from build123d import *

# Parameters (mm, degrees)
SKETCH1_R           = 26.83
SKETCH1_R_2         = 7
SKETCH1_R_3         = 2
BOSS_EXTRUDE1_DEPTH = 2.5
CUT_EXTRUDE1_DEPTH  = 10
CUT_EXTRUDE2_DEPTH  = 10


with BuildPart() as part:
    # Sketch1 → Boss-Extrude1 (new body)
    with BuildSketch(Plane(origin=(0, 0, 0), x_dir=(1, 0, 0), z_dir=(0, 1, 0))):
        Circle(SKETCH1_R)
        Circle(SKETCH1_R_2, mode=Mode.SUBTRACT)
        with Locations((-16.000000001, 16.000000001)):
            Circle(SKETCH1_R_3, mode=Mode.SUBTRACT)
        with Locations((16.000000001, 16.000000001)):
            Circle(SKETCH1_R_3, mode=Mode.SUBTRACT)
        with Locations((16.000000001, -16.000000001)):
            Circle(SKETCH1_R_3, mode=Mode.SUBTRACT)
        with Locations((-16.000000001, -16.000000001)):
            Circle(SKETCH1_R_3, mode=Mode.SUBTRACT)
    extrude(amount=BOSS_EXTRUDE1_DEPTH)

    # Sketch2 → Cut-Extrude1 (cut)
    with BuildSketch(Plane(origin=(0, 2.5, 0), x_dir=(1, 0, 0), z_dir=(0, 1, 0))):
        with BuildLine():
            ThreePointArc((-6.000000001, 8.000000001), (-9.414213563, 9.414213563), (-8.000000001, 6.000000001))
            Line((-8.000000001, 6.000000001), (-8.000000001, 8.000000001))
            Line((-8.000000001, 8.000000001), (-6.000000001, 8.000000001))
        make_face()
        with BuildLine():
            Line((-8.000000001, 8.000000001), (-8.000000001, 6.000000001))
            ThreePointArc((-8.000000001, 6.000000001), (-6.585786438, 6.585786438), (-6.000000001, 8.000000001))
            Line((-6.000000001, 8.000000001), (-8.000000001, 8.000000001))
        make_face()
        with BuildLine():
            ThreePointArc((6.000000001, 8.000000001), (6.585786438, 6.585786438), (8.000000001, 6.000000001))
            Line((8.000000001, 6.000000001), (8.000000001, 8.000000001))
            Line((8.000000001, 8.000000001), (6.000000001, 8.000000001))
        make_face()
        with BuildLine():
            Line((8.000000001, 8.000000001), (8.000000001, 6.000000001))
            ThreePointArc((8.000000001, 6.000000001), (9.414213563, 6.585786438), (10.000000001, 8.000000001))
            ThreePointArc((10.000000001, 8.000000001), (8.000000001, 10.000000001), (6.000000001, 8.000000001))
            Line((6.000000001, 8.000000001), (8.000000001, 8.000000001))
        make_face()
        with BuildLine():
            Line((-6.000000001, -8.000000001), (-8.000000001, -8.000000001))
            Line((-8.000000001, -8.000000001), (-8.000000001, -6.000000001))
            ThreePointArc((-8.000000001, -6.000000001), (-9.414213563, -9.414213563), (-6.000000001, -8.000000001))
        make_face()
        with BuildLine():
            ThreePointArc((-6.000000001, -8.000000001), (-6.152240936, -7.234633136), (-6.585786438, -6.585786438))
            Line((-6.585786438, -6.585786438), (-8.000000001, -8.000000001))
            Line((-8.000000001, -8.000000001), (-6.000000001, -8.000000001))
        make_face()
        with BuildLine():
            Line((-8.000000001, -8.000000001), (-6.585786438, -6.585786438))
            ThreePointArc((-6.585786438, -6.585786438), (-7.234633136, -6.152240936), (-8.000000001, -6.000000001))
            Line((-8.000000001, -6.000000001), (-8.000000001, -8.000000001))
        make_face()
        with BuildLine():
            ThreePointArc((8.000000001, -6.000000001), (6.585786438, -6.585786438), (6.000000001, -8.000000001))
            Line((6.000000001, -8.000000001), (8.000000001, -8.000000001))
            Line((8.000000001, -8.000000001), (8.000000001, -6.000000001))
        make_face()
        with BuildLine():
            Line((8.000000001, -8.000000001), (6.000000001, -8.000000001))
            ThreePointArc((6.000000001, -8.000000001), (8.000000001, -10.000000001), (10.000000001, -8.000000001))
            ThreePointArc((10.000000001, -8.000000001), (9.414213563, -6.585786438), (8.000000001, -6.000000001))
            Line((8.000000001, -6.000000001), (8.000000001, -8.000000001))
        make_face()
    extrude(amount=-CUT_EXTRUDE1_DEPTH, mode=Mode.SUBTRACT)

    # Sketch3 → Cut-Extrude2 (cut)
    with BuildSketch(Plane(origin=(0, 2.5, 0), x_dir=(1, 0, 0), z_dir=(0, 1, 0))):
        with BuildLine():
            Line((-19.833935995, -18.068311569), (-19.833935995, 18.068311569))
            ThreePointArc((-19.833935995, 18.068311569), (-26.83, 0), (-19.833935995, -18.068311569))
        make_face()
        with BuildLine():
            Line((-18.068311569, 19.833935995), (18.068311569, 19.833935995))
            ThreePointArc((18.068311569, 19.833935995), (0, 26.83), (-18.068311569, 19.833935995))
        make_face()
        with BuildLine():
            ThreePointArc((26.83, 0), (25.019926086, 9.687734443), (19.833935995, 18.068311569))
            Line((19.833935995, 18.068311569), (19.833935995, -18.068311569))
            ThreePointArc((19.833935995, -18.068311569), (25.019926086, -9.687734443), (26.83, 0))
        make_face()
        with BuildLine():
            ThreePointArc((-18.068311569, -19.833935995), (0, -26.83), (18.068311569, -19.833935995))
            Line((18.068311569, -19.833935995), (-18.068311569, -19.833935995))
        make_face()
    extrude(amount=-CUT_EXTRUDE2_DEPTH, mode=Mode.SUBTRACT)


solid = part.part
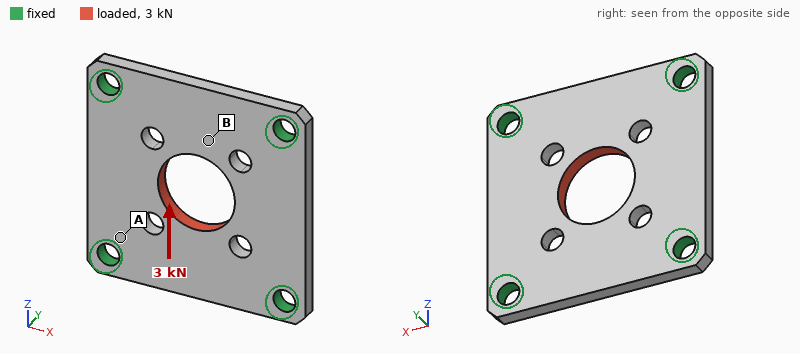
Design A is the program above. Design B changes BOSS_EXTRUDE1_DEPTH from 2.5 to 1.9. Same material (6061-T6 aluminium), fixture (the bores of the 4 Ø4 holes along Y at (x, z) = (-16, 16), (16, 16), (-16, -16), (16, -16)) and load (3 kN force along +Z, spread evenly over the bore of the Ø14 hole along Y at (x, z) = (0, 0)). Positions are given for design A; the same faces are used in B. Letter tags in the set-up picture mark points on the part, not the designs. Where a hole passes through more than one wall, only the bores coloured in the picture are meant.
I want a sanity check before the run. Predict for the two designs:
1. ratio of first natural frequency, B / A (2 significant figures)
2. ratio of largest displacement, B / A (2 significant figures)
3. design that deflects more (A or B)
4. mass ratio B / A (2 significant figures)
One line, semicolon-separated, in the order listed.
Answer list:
0.79; 1.3; B; 0.76
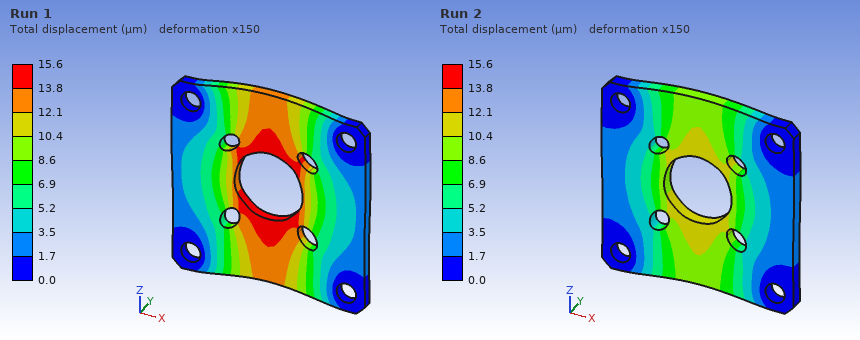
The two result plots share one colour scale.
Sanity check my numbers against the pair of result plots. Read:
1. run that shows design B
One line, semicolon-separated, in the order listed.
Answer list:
Run 1
